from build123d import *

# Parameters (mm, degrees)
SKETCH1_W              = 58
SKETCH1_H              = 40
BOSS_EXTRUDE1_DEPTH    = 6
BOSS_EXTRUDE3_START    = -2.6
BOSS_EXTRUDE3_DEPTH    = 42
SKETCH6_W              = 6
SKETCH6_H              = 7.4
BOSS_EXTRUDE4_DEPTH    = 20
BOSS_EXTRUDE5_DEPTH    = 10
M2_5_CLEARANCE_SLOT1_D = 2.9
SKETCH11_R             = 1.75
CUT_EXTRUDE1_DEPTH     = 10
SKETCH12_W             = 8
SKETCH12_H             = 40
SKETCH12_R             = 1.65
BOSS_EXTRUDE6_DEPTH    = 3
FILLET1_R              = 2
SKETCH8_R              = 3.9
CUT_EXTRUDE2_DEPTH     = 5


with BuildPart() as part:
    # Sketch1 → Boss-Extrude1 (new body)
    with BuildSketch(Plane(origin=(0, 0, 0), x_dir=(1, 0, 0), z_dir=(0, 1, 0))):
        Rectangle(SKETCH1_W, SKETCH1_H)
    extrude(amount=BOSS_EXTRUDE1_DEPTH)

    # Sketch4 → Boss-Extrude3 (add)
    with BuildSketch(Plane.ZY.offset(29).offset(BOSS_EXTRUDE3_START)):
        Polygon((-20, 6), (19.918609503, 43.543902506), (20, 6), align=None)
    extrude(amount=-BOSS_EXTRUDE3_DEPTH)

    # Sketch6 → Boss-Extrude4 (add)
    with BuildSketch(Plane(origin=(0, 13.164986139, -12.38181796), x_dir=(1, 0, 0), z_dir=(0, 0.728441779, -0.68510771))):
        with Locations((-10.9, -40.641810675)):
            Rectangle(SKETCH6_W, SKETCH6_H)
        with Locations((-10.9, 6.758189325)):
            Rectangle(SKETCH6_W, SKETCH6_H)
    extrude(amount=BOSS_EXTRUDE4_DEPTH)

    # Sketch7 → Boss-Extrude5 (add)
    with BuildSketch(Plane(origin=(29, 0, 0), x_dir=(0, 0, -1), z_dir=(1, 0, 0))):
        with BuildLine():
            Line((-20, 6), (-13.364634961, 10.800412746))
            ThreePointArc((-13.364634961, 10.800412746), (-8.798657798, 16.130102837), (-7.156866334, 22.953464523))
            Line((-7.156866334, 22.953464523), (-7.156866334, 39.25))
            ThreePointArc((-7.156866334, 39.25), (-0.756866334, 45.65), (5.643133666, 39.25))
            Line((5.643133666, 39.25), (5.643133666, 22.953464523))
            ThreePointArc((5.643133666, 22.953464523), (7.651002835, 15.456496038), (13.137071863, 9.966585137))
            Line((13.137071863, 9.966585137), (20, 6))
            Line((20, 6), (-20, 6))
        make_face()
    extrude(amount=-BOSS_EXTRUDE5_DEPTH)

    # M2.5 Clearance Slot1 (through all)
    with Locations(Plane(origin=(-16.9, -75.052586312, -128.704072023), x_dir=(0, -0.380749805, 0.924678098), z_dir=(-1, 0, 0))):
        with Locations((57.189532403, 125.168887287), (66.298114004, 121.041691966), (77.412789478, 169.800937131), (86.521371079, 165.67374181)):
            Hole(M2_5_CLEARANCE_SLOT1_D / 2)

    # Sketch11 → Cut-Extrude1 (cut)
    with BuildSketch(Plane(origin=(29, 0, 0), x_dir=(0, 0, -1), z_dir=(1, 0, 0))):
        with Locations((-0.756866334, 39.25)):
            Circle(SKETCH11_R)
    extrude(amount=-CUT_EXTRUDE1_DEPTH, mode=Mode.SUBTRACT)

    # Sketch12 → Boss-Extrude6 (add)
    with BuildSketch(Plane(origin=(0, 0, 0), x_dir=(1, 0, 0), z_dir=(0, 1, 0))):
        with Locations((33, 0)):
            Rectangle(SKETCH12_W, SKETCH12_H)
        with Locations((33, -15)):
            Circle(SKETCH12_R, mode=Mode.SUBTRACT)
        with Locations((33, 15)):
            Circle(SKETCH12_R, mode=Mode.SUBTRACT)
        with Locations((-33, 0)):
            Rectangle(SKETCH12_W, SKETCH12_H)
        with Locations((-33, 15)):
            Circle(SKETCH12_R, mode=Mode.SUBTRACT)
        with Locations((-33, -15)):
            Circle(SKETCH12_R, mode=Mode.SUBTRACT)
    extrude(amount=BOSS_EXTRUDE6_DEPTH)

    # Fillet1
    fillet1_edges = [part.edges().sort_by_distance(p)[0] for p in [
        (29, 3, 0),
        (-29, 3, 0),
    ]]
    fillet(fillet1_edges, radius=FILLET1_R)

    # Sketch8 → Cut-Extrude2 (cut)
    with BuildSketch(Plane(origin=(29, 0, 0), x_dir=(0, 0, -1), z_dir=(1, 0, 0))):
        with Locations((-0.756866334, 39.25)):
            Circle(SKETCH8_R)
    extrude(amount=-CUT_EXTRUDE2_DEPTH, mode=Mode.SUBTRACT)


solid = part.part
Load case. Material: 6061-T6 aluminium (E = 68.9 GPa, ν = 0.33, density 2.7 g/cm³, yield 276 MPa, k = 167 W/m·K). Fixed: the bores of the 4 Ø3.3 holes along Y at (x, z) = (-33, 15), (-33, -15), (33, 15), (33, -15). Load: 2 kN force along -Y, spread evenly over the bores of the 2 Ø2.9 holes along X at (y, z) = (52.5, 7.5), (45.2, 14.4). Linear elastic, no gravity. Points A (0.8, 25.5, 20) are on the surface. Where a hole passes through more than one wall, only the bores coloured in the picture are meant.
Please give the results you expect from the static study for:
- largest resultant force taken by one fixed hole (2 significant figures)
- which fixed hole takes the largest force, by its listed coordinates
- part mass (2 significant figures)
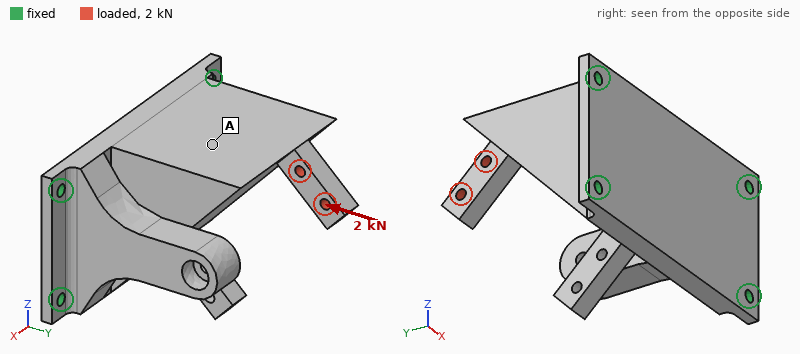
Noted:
1.4 kN
(-33, 15)
150 g
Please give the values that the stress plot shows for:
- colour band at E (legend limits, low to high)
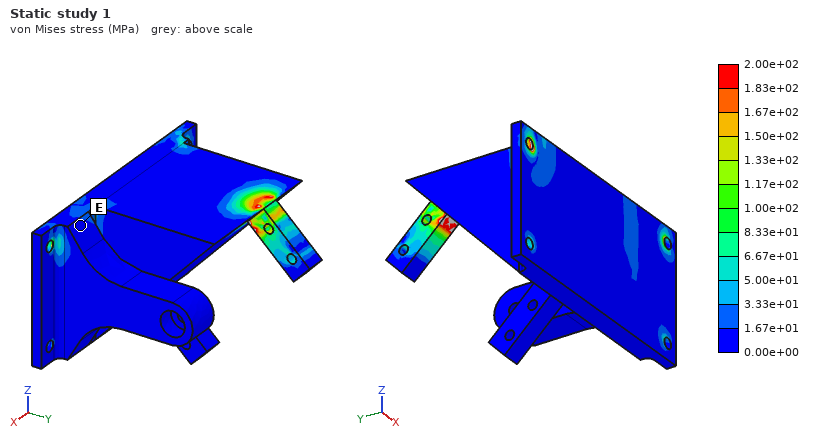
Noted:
0.00e+00 to 1.67e+01 MPa
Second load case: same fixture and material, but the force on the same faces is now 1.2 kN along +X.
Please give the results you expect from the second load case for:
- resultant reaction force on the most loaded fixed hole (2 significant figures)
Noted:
750 N
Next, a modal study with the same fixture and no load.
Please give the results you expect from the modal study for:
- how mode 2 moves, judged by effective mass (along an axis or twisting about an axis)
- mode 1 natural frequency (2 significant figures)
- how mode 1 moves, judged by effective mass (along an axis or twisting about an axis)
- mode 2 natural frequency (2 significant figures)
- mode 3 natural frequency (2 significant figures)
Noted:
along Z
3500 Hz
along Y
4100 Hz
6200 Hz
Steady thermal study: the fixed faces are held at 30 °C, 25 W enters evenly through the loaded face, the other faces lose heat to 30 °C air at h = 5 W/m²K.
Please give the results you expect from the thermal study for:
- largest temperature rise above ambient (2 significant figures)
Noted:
71 K
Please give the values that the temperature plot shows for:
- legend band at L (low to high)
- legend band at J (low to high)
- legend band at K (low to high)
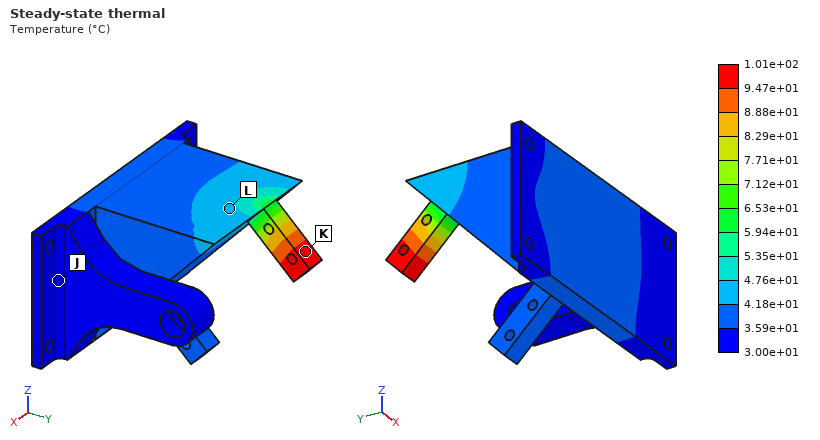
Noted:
4.18e+01 to 4.76e+01 °C
3.00e+01 to 3.59e+01 °C
9.47e+01 to 1.01e+02 °C
